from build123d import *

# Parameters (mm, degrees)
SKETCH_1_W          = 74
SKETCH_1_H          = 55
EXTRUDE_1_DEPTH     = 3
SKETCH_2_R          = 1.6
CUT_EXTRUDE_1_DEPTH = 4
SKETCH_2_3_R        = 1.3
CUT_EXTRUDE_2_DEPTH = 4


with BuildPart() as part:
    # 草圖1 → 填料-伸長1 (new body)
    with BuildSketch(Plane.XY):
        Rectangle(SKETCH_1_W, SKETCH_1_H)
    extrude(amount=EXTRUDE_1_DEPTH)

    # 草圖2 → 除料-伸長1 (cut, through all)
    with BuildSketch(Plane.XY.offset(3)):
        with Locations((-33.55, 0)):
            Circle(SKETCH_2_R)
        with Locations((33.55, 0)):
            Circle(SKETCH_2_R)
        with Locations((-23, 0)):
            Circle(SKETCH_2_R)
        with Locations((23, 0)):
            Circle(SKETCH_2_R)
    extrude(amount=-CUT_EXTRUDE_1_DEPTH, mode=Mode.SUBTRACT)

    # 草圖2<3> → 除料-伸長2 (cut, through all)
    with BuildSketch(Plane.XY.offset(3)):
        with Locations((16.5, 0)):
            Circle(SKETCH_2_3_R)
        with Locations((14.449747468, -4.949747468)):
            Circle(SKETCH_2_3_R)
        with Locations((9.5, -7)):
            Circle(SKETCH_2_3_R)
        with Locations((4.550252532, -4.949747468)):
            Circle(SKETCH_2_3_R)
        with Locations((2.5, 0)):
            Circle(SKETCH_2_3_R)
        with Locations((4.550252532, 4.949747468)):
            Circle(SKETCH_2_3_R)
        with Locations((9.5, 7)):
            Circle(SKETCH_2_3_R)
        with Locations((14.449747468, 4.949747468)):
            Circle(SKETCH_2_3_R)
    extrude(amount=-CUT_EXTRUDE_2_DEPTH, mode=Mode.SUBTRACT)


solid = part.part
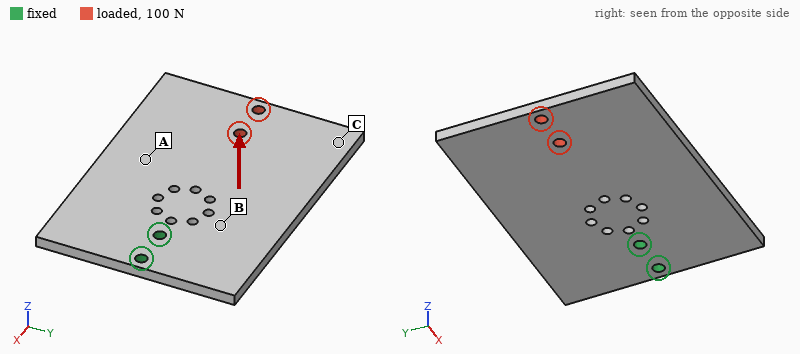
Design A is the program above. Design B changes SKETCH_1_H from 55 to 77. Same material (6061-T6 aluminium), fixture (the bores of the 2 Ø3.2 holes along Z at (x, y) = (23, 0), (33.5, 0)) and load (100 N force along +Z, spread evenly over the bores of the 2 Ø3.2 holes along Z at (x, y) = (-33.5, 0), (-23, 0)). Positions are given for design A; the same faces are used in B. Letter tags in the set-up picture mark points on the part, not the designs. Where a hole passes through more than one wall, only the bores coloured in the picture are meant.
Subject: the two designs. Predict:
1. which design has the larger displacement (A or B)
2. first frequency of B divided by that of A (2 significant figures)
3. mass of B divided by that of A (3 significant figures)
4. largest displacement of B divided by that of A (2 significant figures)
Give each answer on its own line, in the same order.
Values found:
A
0.91
1.41
0.85
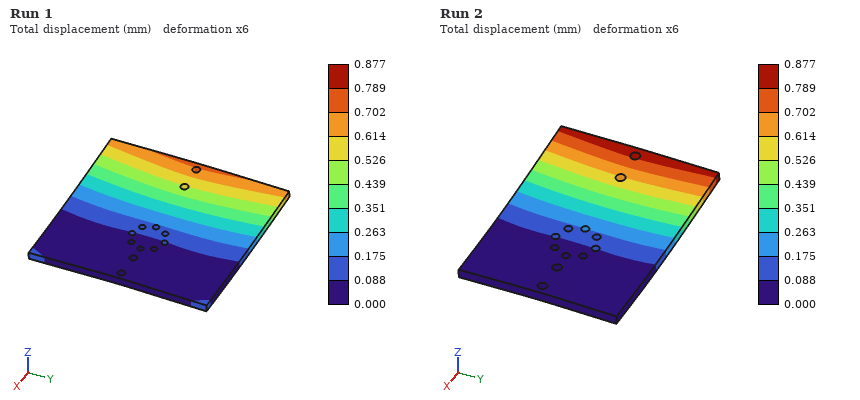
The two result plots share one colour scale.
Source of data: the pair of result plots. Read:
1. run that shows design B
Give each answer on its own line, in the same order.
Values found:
Run 1
